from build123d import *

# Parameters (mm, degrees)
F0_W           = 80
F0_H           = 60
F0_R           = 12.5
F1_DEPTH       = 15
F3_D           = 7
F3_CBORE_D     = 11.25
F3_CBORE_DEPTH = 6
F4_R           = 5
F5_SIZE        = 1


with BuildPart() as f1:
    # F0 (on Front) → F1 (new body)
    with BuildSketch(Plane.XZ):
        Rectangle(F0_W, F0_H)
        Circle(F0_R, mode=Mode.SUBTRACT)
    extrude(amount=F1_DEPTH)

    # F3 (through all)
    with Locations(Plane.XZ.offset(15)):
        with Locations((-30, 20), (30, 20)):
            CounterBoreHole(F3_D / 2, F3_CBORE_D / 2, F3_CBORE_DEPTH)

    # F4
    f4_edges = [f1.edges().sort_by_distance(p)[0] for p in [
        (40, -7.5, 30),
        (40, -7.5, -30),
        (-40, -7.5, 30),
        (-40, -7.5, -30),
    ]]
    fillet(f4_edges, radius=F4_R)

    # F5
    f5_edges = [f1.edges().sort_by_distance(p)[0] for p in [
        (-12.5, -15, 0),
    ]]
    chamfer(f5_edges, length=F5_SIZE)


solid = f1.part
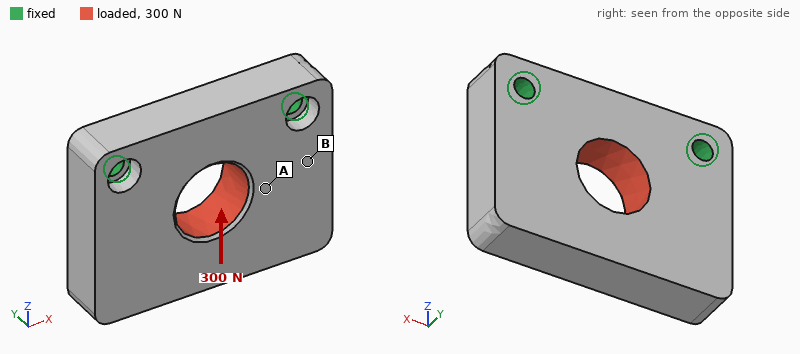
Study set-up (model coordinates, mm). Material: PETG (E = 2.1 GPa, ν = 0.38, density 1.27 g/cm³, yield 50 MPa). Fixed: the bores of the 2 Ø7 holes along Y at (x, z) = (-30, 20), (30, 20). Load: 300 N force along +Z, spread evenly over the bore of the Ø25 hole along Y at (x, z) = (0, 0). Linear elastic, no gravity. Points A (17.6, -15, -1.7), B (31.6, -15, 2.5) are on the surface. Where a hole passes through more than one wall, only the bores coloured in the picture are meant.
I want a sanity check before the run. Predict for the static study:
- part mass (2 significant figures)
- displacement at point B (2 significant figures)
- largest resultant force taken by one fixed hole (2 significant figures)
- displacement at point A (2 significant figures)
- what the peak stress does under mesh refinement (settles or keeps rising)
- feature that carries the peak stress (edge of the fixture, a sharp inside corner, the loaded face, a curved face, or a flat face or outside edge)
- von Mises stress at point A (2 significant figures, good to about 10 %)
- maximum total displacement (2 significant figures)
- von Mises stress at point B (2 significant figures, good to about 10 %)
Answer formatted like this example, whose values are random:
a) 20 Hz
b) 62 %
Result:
a) 79 g
b) 10 µm
c) 150 N
d) 15 µm
e) keeps rising
f) edge of the fixture
g) 0.39 MPa
h) 24 µm
i) 0.25 MPa
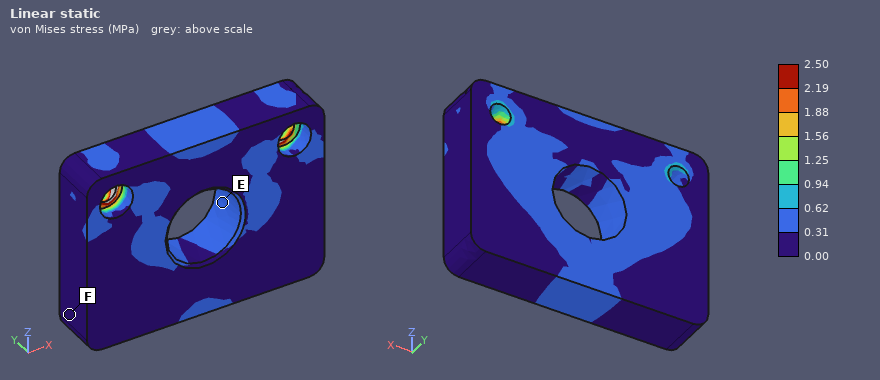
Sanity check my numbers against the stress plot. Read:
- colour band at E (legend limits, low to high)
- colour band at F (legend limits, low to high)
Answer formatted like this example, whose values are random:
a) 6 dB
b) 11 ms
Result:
a) 0.31 to 0.62 MPa
b) 0.00 to 0.31 MPa
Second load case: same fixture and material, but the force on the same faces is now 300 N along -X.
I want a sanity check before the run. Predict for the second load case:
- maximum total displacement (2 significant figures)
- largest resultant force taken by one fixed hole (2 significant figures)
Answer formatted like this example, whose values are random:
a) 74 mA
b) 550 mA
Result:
a) 25 µm
b) 170 N
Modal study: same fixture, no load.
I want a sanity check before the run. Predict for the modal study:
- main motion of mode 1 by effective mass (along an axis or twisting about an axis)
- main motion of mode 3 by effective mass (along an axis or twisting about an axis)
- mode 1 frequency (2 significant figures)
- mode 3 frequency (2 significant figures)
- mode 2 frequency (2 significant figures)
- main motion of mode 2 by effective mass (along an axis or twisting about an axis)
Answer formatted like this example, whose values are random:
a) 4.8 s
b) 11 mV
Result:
a) along Y
b) along X
c) 710 Hz
d) 2200 Hz
e) 1500 Hz
f) twisting about Z
